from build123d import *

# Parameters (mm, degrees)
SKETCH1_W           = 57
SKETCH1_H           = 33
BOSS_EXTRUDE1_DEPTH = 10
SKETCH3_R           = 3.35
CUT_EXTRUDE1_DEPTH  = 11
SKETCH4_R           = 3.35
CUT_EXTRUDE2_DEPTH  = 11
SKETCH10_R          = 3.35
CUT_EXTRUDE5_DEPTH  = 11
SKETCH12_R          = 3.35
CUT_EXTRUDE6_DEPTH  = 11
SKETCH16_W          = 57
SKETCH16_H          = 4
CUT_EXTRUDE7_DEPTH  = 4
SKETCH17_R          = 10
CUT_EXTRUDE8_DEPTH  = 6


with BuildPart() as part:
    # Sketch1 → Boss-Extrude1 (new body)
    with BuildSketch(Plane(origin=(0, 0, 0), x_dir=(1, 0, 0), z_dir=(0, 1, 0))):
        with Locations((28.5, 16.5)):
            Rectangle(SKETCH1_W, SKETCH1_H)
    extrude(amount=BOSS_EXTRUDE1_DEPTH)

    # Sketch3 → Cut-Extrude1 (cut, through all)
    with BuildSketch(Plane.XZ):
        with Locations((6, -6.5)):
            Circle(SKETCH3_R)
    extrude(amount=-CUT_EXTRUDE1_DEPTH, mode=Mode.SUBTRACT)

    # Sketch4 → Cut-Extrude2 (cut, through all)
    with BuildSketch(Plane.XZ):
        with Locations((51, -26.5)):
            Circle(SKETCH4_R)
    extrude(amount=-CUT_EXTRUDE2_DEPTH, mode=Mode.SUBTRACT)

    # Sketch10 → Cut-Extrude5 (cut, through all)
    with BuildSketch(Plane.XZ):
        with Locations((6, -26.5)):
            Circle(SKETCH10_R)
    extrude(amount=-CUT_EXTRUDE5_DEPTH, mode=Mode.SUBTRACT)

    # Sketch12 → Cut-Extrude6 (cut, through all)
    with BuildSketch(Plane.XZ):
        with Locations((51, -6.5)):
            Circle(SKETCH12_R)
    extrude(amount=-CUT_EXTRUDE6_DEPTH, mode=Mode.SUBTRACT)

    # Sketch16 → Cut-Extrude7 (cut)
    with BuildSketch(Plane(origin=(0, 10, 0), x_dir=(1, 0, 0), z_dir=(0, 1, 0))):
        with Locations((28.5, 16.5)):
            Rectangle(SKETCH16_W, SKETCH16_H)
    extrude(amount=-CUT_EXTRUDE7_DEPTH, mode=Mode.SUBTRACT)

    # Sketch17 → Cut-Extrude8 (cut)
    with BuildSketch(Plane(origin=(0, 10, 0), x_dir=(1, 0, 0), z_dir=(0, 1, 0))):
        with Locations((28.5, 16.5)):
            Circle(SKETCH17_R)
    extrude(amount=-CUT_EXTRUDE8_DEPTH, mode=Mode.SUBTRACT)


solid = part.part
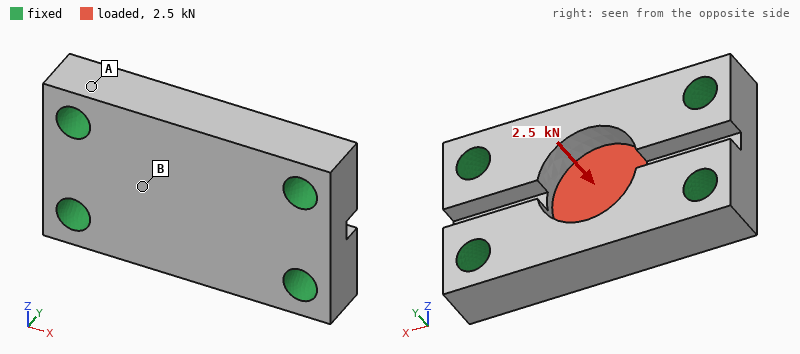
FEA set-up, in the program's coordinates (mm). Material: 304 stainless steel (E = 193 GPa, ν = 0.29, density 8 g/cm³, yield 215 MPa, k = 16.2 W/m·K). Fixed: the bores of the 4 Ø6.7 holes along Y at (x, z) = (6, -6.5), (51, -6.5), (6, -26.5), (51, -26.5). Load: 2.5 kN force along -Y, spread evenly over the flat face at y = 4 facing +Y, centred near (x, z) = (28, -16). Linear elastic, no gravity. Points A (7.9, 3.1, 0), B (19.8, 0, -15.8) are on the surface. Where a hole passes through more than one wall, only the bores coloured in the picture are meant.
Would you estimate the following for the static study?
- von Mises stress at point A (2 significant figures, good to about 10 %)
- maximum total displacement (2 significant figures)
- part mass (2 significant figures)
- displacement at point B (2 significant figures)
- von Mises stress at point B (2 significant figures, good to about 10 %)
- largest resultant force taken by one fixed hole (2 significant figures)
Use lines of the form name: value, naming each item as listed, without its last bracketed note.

von Mises stress at point A: 5.3 MPa
maximum total displacement: 6.0 µm
part mass: 120 g
displacement at point B: 3.3 µm
von Mises stress at point B: 17 MPa
largest resultant force taken by one fixed hole: 670 N
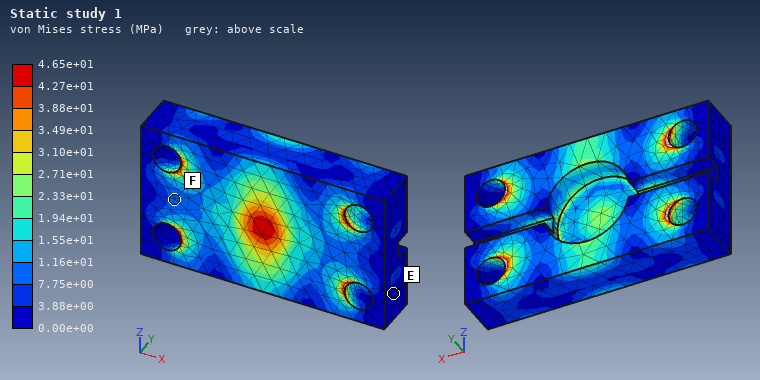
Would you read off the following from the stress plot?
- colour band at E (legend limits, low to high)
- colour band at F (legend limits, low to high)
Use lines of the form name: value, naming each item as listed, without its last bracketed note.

colour band at E: 0.00e+00 to 3.88e+00 MPa
colour band at F: 7.75e+00 to 1.16e+01 MPa
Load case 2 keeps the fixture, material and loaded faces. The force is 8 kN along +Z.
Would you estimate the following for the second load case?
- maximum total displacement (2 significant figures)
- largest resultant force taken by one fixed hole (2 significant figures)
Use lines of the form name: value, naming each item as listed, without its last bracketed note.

maximum total displacement: 7.1 µm
largest resultant force taken by one fixed hole: 2.3 kN
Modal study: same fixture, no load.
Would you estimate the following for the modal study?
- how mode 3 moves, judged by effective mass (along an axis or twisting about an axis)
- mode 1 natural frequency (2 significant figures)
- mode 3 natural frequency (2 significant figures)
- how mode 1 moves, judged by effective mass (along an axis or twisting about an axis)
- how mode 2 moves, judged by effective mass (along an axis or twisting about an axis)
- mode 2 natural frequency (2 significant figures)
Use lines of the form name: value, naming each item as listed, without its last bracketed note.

how mode 3 moves, judged by effective mass: along Z
mode 1 natural frequency: 23 kHz
mode 3 natural frequency: 33 kHz
how mode 1 moves, judged by effective mass: along Y
how mode 2 moves, judged by effective mass: twisting about X
mode 2 natural frequency: 26 kHz
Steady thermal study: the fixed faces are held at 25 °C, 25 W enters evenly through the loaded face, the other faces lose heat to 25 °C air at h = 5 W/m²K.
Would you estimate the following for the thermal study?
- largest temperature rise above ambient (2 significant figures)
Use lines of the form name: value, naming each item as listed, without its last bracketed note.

largest temperature rise above ambient: 78 K
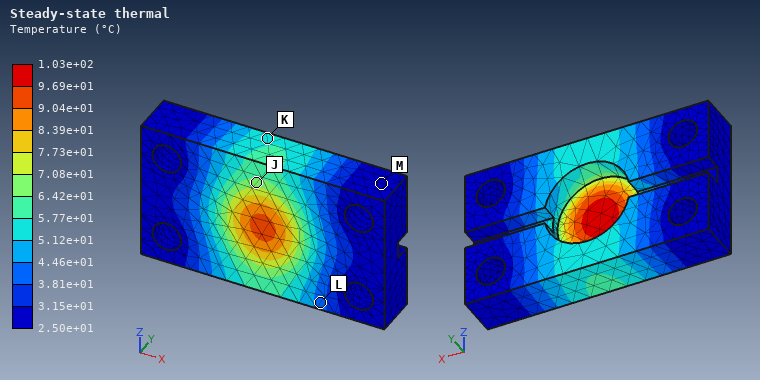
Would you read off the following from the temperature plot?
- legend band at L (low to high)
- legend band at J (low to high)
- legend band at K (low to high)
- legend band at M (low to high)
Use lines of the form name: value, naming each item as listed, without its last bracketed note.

legend band at L: 3.81e+01 to 4.46e+01 °C
legend band at J: 6.42e+01 to 7.08e+01 °C
legend band at K: 5.12e+01 to 5.77e+01 °C
legend band at M: 2.50e+01 to 3.15e+01 °C
